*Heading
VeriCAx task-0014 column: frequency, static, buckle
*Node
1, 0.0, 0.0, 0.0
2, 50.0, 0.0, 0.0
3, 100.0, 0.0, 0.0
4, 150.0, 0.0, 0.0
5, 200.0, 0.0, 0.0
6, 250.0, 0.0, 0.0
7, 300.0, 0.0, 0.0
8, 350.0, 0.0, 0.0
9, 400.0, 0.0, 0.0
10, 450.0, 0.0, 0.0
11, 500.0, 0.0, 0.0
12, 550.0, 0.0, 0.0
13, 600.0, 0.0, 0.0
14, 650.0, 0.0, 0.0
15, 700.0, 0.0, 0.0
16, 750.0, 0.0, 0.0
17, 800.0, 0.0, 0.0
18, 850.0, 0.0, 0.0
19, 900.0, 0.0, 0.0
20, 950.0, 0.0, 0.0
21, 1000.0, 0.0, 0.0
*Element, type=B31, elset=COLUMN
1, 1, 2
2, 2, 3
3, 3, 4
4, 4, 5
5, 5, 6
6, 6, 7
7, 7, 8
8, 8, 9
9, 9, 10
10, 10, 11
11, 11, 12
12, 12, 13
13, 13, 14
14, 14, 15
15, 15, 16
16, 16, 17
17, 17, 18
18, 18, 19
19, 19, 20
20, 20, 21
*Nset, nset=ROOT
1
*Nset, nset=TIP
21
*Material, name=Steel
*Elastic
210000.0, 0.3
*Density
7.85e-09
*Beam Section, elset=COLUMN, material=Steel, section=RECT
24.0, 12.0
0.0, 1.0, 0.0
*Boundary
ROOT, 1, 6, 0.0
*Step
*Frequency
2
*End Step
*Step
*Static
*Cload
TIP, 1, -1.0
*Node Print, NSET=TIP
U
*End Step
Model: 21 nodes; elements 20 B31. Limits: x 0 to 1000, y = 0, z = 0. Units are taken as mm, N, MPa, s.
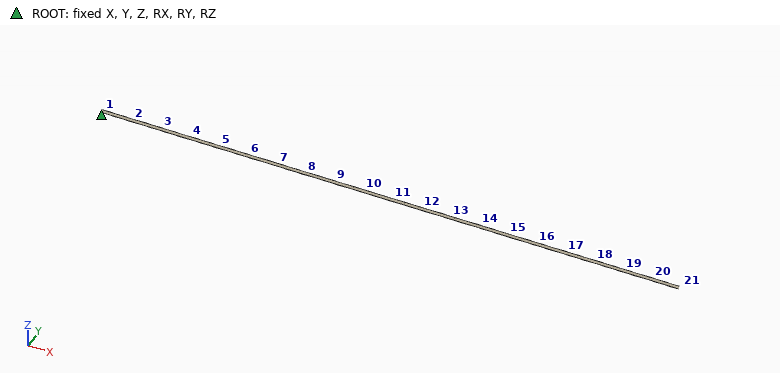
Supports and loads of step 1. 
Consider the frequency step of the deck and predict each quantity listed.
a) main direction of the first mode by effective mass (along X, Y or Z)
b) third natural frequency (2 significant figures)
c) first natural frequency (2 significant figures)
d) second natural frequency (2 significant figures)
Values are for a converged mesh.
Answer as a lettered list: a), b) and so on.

a) along Z
b) 63 Hz
c) 10 Hz
d) 20 Hz
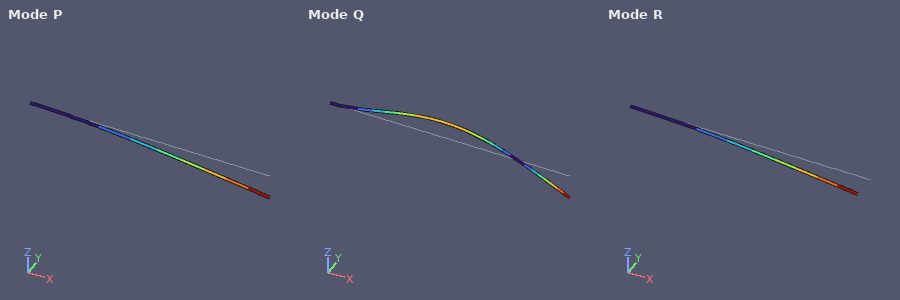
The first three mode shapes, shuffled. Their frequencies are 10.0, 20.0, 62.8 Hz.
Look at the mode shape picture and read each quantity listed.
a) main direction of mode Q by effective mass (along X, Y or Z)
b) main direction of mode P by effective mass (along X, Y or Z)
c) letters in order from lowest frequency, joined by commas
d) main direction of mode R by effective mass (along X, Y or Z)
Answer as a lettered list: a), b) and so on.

a) along Z
b) along Z
c) P, R, Q
d) along Y
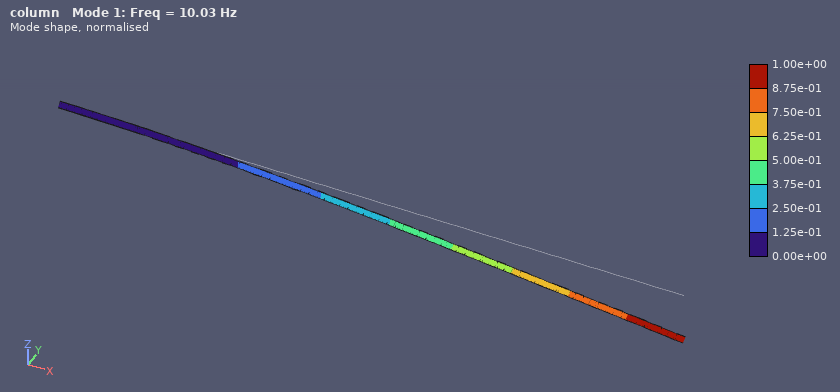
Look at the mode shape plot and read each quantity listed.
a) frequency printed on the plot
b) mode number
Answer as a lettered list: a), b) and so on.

a) 10.03 Hz
b) 1
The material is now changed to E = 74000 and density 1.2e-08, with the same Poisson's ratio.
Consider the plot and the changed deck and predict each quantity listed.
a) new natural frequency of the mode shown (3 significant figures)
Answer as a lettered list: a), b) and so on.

a) 4.81 Hz
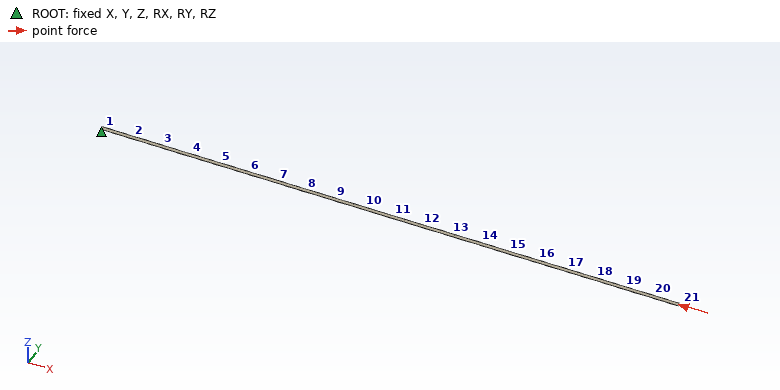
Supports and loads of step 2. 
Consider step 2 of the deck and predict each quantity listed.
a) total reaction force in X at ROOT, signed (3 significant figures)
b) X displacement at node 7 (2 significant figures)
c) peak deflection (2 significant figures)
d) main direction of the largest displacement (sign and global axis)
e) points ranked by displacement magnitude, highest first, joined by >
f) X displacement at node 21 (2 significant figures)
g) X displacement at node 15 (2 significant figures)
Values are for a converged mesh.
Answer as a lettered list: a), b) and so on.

a) 1.00 N
b) -5.0e-06 mm
c) 1.7e-05 mm
d) -X
e) node 21 > node 15 > node 12 > node 10 > node 7
f) -1.7e-05 mm
g) -1.2e-05 mm
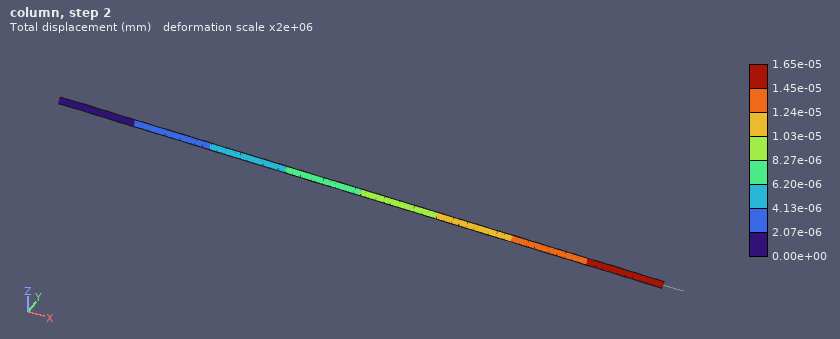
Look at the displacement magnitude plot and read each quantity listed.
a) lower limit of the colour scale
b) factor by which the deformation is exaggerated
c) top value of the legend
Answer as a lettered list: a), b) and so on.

a) 0.00e+00 mm
b) 2e+06
c) 1.65e-05 mm
